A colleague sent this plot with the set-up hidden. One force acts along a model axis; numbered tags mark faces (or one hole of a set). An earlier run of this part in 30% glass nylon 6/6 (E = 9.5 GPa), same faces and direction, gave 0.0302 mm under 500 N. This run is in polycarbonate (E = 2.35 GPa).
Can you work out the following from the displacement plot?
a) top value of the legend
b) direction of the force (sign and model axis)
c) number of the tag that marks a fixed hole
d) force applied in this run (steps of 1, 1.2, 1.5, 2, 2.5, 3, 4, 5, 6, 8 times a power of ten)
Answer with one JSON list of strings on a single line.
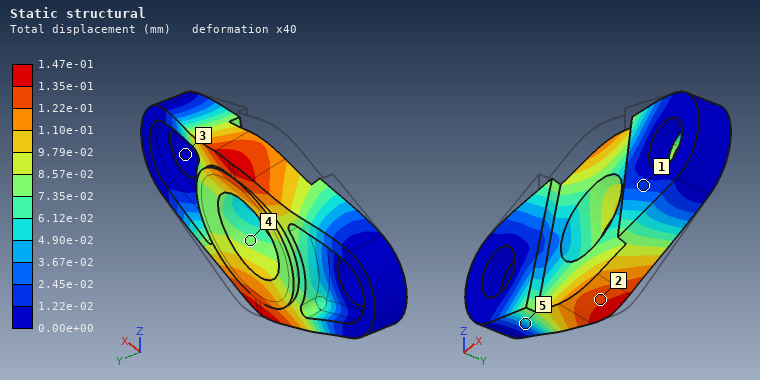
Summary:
["1.47e-01 mm", "-Z", "3", "600 N"]
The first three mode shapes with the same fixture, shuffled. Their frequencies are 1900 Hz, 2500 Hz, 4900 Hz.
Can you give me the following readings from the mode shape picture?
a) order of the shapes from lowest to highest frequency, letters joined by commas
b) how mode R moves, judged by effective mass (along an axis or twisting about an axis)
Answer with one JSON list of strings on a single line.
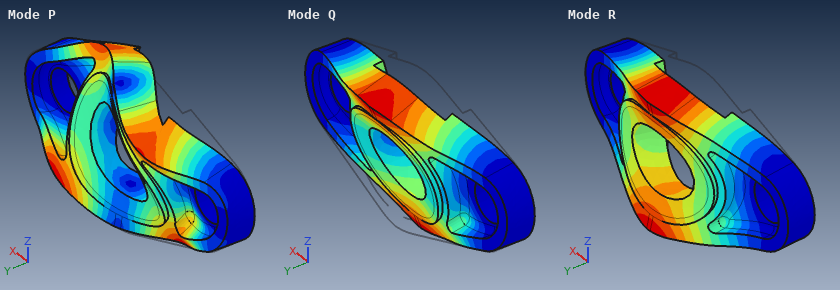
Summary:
["Q, R, P", "along Y"]
